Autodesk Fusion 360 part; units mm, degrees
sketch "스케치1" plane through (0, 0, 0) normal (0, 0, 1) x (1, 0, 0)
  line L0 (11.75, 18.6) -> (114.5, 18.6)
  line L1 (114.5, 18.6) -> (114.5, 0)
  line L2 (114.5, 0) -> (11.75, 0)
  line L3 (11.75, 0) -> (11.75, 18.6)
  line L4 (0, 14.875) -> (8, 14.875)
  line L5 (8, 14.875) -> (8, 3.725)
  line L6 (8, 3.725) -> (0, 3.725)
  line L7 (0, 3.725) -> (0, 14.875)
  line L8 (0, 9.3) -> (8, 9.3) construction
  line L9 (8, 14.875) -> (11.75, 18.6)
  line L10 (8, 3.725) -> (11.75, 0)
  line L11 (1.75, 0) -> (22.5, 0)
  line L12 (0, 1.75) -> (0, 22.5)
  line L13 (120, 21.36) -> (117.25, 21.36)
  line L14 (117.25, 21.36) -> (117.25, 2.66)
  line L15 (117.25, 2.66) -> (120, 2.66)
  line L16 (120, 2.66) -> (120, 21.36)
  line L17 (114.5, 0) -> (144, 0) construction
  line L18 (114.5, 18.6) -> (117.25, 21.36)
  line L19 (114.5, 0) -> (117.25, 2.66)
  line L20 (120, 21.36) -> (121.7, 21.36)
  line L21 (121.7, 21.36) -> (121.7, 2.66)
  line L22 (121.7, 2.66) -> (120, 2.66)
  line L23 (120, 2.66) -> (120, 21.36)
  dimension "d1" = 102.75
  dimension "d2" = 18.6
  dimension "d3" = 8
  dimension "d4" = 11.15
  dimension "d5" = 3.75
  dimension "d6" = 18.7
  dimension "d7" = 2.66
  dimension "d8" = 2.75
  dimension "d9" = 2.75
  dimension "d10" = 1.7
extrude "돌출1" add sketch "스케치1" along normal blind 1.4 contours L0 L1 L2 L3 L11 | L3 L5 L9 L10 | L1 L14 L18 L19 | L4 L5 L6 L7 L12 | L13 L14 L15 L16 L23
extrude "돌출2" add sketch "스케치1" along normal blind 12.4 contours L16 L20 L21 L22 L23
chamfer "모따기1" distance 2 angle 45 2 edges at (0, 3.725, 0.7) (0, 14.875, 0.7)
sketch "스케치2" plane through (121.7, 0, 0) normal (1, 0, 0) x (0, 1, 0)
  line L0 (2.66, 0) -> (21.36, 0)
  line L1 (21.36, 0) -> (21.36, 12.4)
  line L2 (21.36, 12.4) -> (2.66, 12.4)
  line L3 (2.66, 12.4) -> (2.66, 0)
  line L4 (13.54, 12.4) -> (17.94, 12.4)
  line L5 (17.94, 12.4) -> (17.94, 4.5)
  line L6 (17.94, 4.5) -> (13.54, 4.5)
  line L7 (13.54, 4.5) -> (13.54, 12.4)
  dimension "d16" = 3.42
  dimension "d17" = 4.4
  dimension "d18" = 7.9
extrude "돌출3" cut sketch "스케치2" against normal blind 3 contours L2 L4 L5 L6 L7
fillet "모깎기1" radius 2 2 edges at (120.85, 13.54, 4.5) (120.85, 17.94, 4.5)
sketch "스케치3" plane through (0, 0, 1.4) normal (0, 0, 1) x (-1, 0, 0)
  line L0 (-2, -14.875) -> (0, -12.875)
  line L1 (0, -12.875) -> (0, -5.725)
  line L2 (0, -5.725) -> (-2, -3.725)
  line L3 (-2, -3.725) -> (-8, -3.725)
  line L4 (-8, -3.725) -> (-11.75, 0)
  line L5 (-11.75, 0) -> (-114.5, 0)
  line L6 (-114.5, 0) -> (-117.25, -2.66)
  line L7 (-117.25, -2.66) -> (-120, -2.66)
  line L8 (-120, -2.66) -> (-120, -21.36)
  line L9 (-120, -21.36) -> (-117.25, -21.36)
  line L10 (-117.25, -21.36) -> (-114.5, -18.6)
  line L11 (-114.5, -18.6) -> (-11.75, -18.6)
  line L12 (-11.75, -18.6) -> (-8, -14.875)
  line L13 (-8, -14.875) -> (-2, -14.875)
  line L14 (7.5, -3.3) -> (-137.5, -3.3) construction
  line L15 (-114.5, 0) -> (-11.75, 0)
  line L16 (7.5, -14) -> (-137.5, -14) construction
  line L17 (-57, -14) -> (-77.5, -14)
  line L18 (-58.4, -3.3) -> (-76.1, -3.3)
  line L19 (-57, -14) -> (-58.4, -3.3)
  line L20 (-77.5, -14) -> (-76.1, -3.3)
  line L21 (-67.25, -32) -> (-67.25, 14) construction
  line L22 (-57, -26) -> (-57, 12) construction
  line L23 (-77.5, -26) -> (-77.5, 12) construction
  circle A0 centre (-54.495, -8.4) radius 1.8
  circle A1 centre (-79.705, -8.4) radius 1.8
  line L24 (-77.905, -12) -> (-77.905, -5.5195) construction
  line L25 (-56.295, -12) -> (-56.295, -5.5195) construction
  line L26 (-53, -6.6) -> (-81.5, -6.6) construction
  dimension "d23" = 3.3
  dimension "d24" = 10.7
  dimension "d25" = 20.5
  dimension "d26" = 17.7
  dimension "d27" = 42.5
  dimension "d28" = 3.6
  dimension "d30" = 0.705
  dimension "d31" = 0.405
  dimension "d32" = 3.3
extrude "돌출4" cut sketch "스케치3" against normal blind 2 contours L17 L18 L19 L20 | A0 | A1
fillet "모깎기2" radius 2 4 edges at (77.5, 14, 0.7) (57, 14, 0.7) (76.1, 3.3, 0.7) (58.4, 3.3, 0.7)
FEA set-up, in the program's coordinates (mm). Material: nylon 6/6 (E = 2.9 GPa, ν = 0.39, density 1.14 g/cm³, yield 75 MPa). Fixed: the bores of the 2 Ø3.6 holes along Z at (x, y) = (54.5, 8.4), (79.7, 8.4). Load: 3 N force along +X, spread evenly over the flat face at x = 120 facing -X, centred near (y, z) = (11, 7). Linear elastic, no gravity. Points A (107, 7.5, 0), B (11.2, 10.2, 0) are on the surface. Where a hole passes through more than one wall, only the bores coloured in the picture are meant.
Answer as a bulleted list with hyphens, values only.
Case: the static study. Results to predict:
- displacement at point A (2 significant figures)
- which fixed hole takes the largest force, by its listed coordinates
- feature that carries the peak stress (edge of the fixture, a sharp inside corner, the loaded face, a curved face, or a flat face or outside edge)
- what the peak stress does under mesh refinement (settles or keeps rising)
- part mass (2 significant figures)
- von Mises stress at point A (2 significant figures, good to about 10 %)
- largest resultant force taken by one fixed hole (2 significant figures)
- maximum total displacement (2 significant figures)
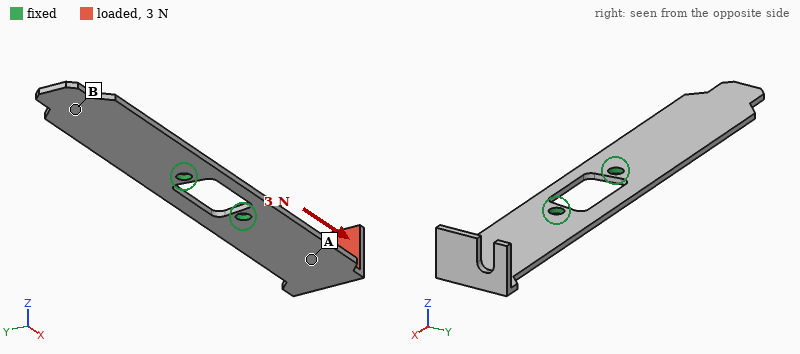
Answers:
- 0.51 mm
- (79.7, 8.4)
- edge of the fixture
- keeps rising
- 3.5 g
- 2.6 MPa
- 2.6 N
- 1.4 mm
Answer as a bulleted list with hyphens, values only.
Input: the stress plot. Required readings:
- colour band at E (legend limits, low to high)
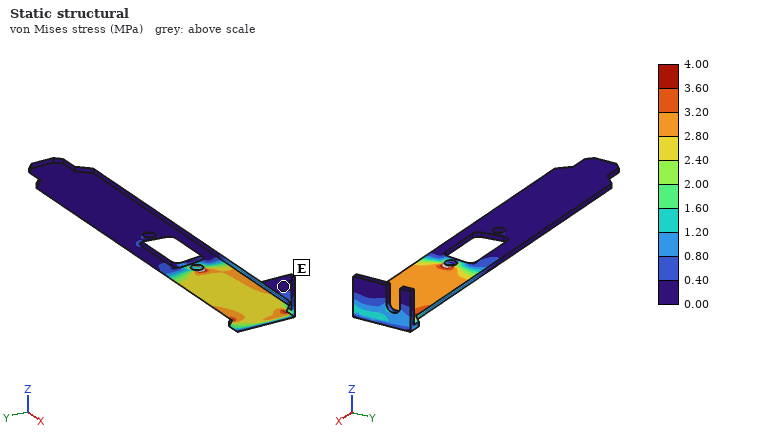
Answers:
- 0.00 to 0.40 MPa
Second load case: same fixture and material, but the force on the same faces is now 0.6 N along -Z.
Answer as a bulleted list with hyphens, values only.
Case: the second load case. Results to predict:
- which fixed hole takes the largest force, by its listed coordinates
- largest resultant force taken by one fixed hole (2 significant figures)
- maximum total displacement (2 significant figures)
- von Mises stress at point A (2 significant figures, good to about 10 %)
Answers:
- (79.7, 8.4)
- 0.72 N
- 1.2 mm
- 1.3 MPa
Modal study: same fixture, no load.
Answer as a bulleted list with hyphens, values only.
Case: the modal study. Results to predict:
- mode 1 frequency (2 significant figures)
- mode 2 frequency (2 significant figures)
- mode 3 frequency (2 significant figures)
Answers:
- 140 Hz
- 150 Hz
- 530 Hz
